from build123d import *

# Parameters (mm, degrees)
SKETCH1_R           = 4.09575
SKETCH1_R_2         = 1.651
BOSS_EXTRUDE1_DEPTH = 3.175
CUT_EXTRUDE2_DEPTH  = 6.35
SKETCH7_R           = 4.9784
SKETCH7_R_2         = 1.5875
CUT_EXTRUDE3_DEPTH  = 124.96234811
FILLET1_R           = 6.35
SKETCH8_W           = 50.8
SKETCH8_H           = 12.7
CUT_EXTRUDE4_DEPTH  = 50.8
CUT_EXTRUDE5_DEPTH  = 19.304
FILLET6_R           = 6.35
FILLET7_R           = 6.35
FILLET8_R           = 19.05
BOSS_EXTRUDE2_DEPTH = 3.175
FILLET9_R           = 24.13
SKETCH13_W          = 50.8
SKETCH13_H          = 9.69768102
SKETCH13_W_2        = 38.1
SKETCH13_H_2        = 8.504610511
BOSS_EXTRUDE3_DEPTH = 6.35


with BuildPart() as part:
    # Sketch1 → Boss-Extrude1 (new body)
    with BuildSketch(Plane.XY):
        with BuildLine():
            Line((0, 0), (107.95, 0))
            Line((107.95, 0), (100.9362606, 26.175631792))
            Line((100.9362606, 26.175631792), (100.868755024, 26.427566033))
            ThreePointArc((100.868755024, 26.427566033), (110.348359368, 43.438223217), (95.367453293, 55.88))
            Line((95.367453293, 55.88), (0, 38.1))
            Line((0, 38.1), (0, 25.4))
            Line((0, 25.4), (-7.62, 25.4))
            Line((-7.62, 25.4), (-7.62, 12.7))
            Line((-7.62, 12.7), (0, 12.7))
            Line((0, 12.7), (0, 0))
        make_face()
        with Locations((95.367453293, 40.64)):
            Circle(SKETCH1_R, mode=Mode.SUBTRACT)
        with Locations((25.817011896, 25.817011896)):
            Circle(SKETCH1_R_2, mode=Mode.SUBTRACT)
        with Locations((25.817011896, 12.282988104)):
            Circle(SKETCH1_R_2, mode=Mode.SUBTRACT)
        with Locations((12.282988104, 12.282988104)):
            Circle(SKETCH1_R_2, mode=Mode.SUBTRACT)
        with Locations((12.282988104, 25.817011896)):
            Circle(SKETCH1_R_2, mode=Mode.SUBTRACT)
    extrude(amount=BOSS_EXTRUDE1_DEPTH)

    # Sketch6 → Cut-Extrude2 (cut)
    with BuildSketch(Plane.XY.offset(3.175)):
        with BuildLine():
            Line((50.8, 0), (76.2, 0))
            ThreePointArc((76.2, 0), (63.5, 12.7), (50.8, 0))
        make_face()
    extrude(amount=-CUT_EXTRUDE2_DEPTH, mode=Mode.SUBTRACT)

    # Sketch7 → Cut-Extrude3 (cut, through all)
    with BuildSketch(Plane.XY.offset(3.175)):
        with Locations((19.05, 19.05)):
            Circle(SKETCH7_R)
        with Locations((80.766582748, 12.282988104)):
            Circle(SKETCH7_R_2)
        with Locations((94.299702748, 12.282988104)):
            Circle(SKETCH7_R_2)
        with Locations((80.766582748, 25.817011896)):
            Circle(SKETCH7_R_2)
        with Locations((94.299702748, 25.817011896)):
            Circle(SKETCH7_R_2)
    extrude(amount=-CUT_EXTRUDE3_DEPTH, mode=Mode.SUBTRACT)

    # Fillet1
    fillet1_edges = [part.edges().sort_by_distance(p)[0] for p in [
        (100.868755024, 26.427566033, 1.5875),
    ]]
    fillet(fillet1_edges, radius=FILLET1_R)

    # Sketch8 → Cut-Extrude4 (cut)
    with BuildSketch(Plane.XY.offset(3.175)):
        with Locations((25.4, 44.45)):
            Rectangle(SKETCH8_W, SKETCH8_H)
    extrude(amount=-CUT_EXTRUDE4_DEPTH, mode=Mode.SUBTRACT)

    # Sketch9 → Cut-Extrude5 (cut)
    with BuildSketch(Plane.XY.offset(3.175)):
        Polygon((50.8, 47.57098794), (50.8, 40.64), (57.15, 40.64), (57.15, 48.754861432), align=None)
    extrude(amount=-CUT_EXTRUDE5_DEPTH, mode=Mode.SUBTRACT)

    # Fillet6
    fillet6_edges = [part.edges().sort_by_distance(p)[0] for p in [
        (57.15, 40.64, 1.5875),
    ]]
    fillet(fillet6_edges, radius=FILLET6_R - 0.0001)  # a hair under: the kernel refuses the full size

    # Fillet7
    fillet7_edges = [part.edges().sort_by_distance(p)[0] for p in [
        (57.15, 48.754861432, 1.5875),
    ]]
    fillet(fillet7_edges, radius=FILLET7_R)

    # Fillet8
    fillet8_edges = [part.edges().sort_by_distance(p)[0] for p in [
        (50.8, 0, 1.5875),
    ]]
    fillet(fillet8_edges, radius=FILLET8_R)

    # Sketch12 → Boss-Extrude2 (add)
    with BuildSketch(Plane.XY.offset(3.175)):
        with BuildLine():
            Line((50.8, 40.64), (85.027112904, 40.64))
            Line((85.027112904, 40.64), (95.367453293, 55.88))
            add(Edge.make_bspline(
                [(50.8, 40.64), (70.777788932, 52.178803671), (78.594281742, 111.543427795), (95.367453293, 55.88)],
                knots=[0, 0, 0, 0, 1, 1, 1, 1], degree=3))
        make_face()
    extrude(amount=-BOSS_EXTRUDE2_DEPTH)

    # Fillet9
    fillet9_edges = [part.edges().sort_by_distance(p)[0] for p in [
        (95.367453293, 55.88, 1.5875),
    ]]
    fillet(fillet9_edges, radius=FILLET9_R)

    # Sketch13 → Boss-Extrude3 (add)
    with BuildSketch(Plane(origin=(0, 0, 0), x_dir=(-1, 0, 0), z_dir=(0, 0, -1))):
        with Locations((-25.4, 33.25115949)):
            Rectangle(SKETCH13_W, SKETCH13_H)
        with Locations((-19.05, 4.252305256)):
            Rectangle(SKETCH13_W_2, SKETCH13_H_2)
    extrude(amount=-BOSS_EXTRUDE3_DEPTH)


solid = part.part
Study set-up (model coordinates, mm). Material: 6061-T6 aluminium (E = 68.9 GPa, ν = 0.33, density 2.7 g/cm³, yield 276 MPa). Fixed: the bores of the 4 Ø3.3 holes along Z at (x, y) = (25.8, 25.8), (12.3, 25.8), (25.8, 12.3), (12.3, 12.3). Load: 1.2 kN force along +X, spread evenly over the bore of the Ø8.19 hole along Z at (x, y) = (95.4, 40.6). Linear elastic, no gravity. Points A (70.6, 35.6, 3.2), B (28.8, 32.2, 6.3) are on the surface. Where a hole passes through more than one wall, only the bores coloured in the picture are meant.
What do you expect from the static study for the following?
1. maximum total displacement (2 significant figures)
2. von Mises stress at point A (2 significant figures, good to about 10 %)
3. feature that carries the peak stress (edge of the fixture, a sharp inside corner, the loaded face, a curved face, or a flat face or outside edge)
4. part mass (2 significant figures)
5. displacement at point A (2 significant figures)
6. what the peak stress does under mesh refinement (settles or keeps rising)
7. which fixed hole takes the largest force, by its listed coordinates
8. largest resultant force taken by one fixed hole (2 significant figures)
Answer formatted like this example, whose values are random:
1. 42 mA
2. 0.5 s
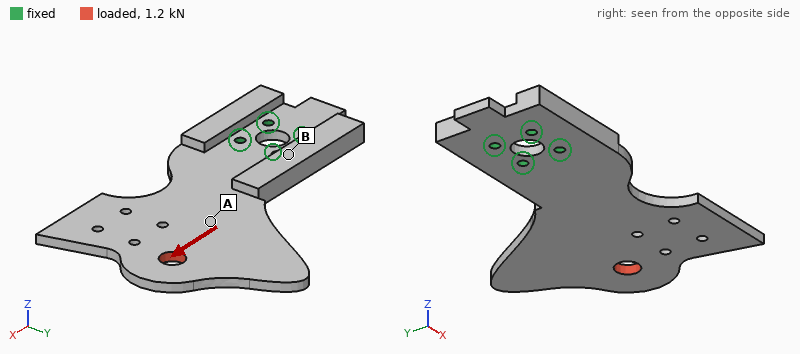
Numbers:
1. 0.20 mm
2. 20 MPa
3. edge of the fixture
4. 50 g
5. 0.087 mm
6. keeps rising
7. (25.8, 25.8)
8. 1.3 kN
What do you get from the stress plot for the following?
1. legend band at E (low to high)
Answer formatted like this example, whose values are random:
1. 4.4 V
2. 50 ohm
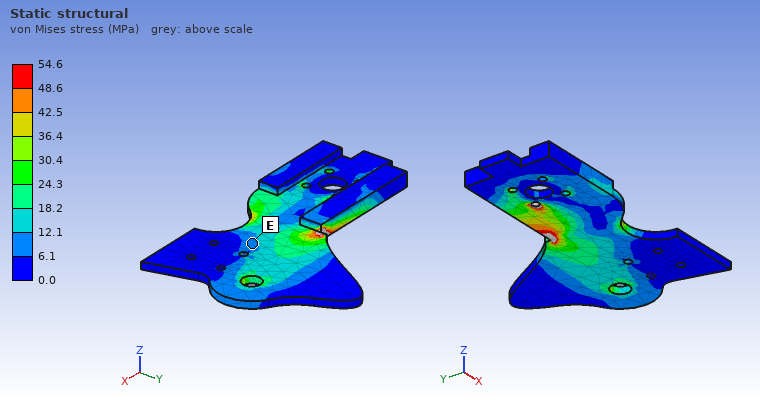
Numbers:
1. 6.1 to 12.1 MPa
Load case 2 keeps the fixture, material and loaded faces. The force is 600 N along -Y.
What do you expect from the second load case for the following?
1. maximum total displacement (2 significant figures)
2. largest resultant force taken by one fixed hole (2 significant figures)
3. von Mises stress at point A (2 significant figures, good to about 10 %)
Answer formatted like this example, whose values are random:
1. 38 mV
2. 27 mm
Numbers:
1. 0.23 mm
2. 1.5 kN
3. 16 MPa
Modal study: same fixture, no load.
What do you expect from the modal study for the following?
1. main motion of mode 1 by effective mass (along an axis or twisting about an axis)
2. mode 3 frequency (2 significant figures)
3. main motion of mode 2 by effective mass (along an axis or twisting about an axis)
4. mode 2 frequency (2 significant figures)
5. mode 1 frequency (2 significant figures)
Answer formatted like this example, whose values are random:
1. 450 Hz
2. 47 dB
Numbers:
1. along Z
2. 2400 Hz
3. twisting about X
4. 850 Hz
5. 420 Hz
